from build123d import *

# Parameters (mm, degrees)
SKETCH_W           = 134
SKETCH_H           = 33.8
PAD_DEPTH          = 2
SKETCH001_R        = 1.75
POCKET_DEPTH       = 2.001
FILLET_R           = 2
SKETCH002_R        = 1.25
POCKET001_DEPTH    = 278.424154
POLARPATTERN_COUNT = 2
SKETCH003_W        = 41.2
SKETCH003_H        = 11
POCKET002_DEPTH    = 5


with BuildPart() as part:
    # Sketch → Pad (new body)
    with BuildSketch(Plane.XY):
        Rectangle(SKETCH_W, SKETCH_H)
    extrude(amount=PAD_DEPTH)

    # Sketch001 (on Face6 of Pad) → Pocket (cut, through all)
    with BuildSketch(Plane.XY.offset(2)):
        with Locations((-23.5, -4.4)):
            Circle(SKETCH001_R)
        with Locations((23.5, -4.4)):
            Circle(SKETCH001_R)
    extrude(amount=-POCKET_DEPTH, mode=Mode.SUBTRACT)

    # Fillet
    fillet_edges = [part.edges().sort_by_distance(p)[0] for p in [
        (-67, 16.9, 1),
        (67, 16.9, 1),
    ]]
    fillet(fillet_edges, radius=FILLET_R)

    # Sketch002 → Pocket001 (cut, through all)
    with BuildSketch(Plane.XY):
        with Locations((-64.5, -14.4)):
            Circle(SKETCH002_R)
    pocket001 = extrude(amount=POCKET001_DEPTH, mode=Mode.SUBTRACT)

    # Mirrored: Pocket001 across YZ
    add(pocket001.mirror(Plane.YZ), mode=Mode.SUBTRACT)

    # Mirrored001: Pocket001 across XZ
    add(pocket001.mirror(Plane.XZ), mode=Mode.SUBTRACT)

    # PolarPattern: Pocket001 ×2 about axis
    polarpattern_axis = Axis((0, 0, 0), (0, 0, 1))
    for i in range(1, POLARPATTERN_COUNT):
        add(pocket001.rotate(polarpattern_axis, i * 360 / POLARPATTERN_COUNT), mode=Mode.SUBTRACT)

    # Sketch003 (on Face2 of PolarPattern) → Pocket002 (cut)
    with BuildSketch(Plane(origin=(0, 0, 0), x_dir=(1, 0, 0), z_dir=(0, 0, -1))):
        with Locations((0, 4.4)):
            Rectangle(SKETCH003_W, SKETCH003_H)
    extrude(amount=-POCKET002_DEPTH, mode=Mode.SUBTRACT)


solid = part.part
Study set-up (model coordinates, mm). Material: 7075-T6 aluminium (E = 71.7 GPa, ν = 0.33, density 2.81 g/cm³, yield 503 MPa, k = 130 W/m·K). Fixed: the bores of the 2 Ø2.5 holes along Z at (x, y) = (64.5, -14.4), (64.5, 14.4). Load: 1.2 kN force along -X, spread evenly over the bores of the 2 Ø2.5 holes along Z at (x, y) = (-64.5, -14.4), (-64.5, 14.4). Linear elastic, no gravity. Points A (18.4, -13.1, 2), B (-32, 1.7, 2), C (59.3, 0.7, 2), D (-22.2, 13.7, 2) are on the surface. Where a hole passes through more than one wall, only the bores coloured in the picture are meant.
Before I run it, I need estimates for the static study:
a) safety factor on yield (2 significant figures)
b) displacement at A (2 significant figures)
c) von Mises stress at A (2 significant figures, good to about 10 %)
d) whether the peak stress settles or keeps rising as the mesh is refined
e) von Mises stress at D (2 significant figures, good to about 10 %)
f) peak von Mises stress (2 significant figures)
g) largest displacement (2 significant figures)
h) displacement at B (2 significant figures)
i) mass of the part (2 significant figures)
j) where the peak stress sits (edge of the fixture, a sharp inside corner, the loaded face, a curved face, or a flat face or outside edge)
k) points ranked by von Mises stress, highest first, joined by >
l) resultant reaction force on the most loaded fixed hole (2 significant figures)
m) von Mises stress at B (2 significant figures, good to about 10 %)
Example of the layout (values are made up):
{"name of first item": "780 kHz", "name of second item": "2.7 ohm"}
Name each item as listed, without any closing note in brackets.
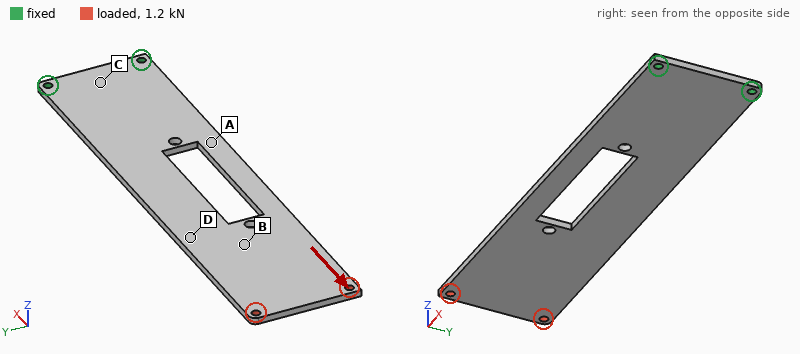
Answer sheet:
{"safety factor on yield": "3.4", "displacement at A": "17 µm", "von Mises stress at A": "31 MPa", "whether the peak stress settles or keeps rising as the mesh is refined": "settles", "von Mises stress at D": "20 MPa", "peak von Mises stress": "150 MPa", "largest displacement": "63 µm", "displacement at B": "36 µm", "mass of the part": "23 g", "where the peak stress sits": "the loaded face", "points ranked by von Mises stress, highest first, joined by >": "A > D > B > C", "resultant reaction force on the most loaded fixed hole": "630 N", "von Mises stress at B": "15 MPa"}
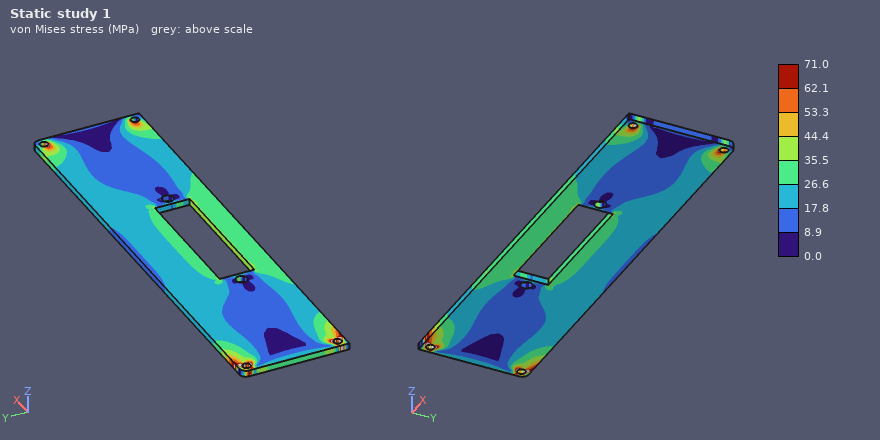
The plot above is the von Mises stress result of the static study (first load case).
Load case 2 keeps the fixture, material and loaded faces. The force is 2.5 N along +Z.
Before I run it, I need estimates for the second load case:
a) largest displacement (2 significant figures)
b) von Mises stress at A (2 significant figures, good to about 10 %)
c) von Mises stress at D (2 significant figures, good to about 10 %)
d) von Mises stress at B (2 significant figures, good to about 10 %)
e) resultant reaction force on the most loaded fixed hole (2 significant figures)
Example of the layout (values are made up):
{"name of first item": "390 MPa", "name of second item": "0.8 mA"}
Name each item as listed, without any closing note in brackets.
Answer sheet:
{"largest displacement": "1.4 mm", "von Mises stress at A": "15 MPa", "von Mises stress at D": "6.3 MPa", "von Mises stress at B": "3.5 MPa", "resultant reaction force on the most loaded fixed hole": "1.3 N"}
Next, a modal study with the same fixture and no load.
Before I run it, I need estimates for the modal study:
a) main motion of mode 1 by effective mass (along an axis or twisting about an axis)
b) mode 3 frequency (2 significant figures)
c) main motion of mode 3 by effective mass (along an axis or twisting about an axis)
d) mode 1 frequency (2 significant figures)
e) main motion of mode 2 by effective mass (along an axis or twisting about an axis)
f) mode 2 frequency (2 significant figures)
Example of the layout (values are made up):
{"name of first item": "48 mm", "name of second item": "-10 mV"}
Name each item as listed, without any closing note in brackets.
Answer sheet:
{"main motion of mode 1 by effective mass": "along Z", "mode 3 frequency": "670 Hz", "main motion of mode 3 by effective mass": "twisting about X", "mode 1 frequency": "89 Hz", "main motion of mode 2 by effective mass": "along Z", "mode 2 frequency": "560 Hz"}
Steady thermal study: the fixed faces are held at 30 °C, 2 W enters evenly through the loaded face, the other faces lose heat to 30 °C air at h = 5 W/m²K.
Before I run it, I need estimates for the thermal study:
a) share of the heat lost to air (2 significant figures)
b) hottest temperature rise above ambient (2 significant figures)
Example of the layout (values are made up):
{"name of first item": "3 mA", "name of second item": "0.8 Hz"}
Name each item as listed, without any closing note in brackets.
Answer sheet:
{"share of the heat lost to air": "31 %", "hottest temperature rise above ambient": "30 K"}
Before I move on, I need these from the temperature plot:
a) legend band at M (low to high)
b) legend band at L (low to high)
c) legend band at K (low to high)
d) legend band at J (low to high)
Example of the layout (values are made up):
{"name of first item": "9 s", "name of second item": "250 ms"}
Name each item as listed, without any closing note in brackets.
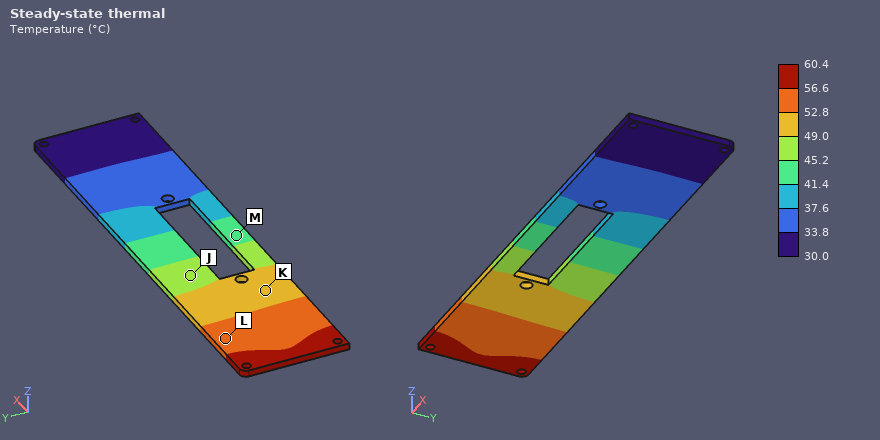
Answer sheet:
{"legend band at M": "41.4 to 45.2 °C", "legend band at L": "52.8 to 56.6 °C", "legend band at K": "49.0 to 52.8 °C", "legend band at J": "45.2 to 49.0 °C"}
